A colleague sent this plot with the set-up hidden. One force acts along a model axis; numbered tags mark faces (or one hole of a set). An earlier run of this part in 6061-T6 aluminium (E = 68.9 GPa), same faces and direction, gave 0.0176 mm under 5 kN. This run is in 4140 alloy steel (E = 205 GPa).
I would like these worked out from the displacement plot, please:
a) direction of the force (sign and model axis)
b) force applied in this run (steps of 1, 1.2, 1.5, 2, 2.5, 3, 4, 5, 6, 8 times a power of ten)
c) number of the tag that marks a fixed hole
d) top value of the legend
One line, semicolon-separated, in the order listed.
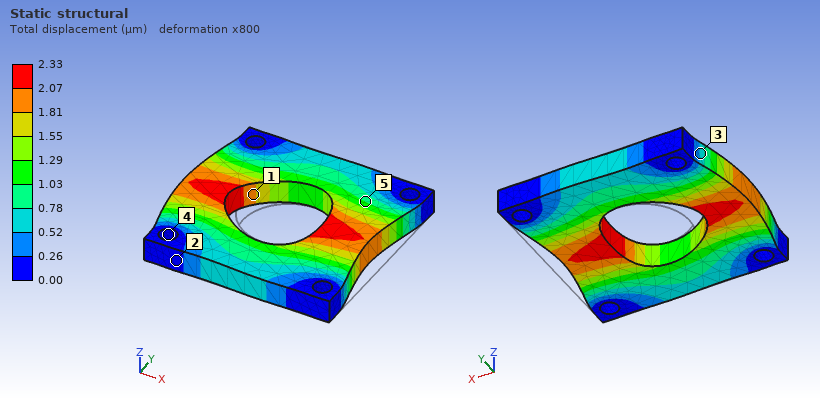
-X; 2 kN; 4; 2.33 µm
